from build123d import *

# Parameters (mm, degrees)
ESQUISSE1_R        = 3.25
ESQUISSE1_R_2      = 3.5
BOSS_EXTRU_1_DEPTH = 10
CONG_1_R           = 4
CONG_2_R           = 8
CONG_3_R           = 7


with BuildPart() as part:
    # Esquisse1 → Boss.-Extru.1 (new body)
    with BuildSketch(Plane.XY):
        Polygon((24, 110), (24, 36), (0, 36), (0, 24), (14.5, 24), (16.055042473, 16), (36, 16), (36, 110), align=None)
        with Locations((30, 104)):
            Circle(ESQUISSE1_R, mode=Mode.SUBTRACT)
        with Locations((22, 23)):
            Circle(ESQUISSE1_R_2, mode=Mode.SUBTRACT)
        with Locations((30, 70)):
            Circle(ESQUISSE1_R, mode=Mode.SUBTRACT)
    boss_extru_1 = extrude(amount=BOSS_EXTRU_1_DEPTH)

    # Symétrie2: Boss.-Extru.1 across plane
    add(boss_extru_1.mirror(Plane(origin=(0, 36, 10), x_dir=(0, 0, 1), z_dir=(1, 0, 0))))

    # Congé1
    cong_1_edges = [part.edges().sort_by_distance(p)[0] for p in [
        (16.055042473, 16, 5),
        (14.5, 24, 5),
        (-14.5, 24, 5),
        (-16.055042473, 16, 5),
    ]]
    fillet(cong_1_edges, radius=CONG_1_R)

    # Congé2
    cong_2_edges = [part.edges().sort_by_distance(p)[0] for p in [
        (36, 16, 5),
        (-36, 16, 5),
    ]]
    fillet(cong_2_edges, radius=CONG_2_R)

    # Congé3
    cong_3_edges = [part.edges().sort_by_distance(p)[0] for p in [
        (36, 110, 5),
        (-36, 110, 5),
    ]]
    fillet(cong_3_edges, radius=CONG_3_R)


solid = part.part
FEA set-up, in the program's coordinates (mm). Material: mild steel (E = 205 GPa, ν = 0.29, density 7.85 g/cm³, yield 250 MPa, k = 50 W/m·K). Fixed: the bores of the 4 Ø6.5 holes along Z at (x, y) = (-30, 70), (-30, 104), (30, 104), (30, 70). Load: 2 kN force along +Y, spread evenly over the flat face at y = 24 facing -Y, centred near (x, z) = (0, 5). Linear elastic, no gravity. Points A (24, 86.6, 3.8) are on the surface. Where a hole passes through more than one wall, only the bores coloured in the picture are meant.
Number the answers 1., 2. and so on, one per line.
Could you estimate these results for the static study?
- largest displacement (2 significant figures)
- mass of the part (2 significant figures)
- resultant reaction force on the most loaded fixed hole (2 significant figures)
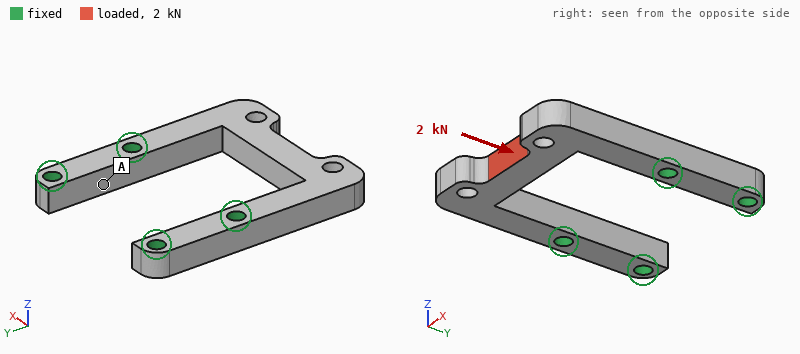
1. 14 µm
2. 210 g
3. 1.1 kN
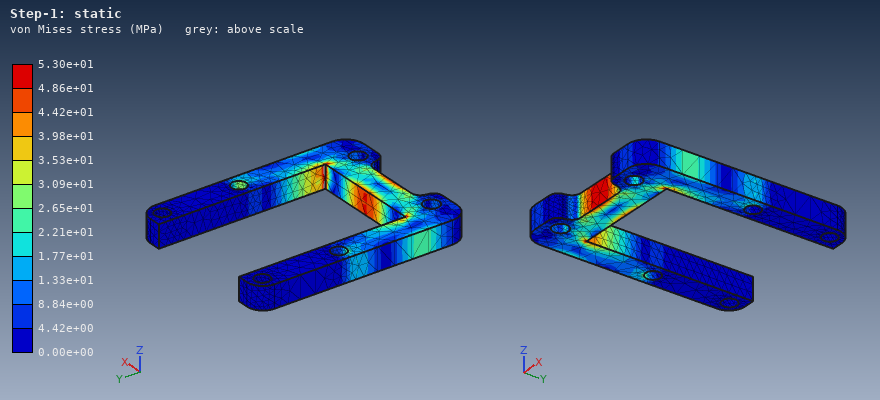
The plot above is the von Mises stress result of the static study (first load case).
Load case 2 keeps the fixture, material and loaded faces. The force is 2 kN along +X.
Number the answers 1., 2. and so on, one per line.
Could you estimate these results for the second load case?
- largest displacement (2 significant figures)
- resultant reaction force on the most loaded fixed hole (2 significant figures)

1. 30 µm
2. 1.3 kN
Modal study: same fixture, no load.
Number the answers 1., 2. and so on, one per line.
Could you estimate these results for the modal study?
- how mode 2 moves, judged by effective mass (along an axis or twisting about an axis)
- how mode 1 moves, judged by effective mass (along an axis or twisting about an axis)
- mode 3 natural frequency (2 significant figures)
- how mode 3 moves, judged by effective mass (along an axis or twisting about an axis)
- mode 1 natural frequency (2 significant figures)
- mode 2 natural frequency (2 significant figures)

1. twisting about Y
2. along Z
3. 4200 Hz
4. along X
5. 2100 Hz
6. 4000 Hz
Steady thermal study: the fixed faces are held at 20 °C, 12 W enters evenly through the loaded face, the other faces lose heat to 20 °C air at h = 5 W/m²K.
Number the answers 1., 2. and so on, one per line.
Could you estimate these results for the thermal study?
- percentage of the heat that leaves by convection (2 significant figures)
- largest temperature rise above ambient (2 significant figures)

1. 8.4 %
2. 57 K
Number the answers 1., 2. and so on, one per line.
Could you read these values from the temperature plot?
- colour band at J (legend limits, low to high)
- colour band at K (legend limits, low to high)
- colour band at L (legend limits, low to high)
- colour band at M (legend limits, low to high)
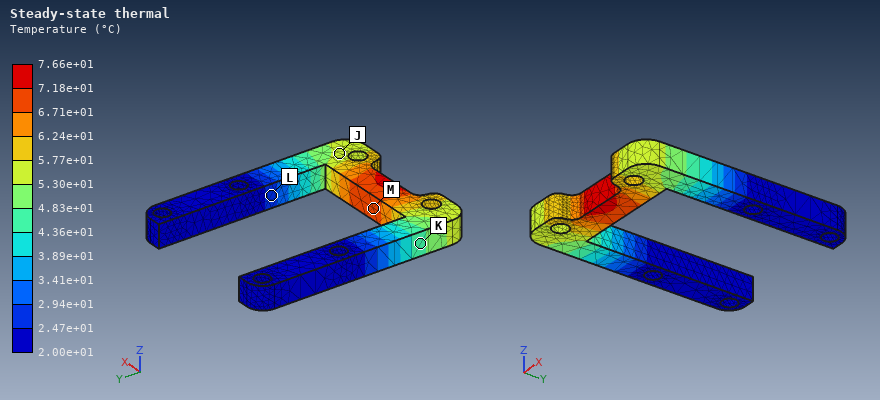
1. 5.30e+01 to 5.77e+01 °C
2. 4.36e+01 to 4.83e+01 °C
3. 2.47e+01 to 2.94e+01 °C
4. 6.71e+01 to 7.18e+01 °C
